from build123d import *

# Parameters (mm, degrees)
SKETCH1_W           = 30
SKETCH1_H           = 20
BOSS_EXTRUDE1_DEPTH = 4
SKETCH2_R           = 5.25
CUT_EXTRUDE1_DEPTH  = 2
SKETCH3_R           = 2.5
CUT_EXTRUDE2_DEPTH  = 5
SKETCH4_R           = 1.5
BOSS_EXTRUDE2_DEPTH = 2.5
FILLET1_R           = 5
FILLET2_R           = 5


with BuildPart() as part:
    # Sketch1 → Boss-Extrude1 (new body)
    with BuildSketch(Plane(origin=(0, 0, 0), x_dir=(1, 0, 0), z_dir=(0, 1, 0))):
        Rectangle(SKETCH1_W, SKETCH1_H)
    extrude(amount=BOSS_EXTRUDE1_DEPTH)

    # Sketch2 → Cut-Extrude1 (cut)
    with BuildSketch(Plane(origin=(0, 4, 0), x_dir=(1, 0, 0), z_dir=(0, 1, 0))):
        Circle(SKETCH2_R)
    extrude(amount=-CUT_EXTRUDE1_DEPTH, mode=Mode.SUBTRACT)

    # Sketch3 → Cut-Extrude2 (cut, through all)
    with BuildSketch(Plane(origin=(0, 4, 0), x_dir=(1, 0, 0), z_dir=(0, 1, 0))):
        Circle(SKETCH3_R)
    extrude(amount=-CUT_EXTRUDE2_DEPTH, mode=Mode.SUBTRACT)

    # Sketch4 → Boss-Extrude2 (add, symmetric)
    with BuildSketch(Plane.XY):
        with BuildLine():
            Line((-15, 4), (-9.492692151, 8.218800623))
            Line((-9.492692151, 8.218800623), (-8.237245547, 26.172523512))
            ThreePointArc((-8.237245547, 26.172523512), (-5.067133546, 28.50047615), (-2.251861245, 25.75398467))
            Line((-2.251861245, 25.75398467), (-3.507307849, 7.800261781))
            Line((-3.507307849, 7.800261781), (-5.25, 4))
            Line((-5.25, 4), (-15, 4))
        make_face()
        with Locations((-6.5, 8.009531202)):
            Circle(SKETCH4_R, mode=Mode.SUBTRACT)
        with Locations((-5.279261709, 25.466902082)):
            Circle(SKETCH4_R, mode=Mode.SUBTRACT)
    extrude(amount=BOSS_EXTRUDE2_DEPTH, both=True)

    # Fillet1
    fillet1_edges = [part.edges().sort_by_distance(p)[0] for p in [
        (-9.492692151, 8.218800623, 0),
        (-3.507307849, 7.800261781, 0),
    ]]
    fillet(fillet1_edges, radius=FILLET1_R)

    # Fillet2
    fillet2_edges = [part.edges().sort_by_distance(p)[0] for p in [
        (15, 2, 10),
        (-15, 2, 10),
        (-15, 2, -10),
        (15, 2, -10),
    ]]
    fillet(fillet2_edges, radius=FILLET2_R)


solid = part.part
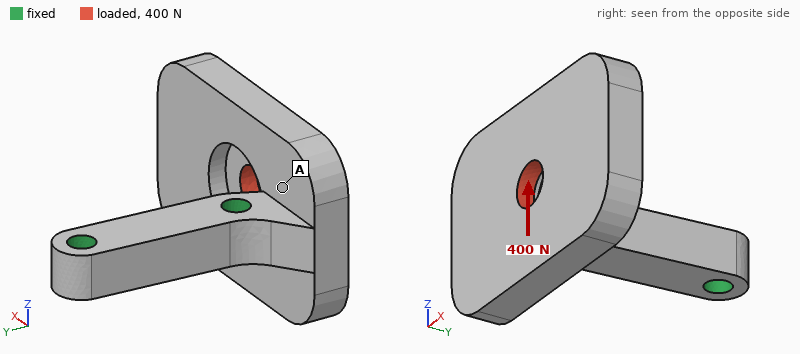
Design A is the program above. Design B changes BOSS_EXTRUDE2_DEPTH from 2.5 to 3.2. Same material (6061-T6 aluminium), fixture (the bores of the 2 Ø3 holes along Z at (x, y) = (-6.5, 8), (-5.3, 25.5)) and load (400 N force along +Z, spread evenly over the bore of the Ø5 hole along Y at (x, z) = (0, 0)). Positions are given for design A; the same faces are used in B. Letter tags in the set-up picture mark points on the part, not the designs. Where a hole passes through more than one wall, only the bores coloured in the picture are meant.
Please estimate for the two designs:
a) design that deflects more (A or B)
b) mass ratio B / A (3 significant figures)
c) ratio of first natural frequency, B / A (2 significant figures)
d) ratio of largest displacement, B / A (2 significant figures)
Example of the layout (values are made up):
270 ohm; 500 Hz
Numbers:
A; 1.07; 1.1; 0.65
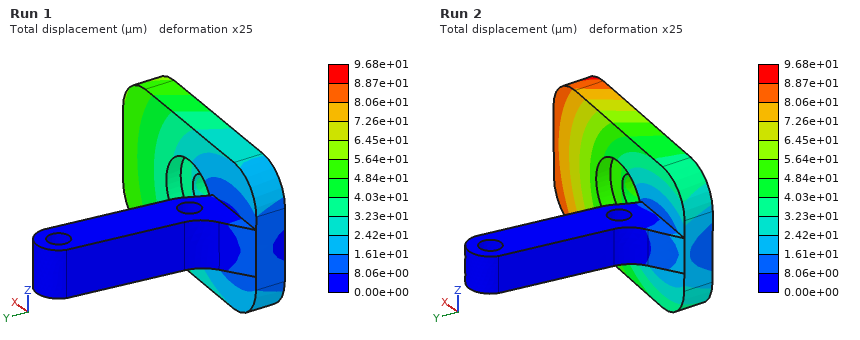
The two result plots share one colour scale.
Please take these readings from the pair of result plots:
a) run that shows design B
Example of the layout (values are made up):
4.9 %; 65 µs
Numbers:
Run 1
